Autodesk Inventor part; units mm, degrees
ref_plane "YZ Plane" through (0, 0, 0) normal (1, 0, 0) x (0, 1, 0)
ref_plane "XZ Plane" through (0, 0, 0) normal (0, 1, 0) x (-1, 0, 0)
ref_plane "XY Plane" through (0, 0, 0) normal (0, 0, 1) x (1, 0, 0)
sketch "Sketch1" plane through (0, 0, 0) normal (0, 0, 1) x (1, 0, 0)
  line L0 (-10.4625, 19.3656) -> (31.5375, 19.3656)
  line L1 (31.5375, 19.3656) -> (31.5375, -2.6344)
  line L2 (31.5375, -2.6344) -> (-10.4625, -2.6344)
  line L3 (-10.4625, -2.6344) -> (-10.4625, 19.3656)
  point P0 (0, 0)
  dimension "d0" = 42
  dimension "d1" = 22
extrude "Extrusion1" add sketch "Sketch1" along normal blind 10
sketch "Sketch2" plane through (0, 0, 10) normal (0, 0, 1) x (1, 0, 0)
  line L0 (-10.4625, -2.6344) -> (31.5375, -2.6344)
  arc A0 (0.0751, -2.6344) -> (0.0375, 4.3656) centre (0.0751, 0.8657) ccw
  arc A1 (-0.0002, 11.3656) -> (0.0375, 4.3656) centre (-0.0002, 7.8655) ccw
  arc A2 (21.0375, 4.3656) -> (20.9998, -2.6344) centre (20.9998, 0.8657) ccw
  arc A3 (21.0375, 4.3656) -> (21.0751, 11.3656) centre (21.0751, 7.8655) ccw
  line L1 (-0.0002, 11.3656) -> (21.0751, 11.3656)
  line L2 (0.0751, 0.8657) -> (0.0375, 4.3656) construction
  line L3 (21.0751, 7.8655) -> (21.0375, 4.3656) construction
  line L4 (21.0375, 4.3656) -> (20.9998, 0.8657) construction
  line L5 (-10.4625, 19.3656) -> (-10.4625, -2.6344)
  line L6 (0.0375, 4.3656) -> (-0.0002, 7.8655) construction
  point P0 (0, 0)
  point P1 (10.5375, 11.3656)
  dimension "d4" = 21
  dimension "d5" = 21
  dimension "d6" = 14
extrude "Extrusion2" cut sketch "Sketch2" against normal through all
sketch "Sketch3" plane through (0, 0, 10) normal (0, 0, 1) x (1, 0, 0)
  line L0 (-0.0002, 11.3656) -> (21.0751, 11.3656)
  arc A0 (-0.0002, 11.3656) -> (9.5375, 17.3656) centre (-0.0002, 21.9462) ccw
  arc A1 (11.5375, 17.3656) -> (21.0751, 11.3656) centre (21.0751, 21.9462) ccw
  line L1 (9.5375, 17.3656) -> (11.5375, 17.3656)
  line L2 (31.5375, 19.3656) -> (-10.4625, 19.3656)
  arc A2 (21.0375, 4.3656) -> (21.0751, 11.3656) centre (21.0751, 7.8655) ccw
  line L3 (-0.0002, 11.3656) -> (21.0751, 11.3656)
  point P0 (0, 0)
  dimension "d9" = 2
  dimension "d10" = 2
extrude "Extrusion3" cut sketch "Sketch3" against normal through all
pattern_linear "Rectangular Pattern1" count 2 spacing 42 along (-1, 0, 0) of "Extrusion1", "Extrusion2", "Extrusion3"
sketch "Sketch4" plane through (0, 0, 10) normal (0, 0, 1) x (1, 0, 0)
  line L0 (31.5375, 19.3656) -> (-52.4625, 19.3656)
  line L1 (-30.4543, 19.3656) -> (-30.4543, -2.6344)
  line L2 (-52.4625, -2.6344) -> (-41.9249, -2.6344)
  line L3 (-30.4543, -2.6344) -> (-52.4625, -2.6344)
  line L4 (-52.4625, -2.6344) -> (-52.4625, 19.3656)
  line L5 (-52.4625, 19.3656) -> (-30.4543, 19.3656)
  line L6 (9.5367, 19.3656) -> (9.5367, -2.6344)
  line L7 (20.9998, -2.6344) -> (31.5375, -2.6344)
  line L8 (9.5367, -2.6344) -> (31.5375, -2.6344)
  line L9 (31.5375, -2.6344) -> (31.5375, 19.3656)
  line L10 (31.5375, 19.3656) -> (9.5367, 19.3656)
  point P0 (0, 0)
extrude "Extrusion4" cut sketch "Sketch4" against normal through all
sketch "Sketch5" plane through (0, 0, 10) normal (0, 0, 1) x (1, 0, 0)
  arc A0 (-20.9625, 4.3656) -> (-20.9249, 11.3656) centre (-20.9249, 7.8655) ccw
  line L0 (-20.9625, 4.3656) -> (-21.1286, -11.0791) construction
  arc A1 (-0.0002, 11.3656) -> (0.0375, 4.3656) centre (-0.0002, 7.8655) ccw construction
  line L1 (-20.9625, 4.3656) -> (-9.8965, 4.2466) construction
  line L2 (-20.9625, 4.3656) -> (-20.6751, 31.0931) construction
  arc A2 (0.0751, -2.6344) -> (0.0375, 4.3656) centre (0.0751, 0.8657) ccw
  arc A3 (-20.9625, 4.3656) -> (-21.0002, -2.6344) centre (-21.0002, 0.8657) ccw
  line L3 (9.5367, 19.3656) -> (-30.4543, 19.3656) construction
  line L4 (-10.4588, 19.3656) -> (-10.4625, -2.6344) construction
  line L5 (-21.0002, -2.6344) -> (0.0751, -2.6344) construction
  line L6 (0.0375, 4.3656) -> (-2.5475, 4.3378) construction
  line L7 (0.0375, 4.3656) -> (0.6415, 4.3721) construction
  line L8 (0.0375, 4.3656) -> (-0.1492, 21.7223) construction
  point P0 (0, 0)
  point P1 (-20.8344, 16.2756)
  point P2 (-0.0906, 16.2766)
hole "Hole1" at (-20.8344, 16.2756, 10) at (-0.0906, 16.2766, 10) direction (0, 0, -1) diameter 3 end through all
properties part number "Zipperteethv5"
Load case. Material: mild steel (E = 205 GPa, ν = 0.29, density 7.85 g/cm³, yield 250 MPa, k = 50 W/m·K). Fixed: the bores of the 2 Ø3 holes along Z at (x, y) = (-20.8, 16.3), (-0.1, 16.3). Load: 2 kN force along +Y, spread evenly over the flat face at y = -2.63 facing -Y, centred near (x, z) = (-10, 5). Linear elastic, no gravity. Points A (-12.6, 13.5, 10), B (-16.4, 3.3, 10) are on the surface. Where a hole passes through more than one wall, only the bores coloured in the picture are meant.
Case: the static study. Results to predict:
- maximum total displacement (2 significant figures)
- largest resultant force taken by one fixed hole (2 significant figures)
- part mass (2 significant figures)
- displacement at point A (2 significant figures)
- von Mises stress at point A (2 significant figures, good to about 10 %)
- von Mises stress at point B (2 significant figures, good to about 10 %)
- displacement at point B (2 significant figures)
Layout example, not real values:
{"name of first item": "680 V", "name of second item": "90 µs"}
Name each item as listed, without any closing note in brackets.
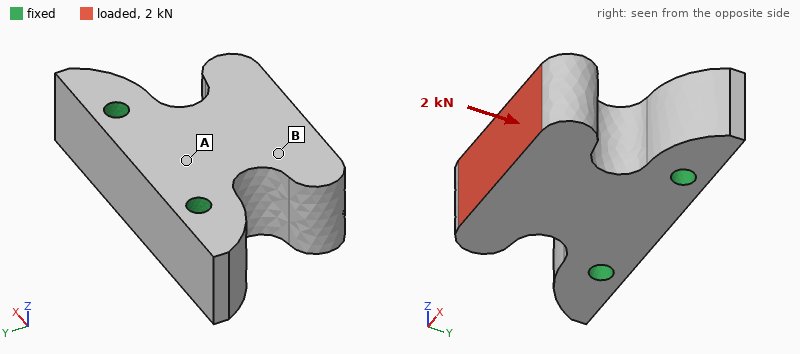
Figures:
{"maximum total displacement": "2.1 µm", "largest resultant force taken by one fixed hole": "1.1 kN", "part mass": "45 g", "displacement at point A": "1.1 µm", "von Mises stress at point A": "5.9 MPa", "von Mises stress at point B": "14 MPa", "displacement at point B": "1.5 µm"}
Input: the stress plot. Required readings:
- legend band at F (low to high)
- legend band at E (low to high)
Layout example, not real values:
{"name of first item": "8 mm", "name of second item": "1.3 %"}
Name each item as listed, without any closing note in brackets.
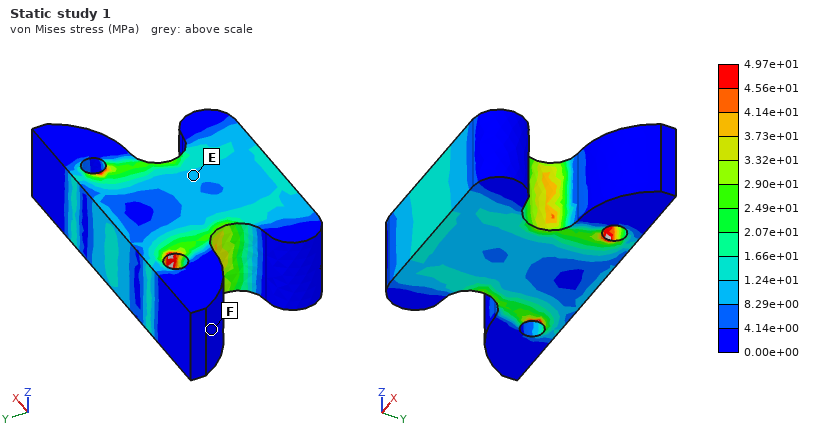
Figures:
{"legend band at F": "0.00e+00 to 4.14e+00 MPa", "legend band at E": "8.29e+00 to 1.24e+01 MPa"}
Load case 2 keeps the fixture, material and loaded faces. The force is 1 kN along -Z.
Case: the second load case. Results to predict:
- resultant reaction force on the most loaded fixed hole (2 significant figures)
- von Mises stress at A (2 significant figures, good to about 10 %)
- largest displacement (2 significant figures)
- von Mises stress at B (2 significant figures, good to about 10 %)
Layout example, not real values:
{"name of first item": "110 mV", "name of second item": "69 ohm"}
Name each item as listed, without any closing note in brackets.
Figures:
{"resultant reaction force on the most loaded fixed hole": "500 N", "von Mises stress at A": "31 MPa", "largest displacement": "16 µm", "von Mises stress at B": "20 MPa"}
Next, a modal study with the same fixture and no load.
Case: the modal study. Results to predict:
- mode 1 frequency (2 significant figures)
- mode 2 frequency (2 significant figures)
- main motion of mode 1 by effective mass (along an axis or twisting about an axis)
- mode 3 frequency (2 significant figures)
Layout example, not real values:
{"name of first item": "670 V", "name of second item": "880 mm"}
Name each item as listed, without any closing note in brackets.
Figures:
{"mode 1 frequency": "12 kHz", "mode 2 frequency": "21 kHz", "main motion of mode 1 by effective mass": "along Z", "mode 3 frequency": "22 kHz"}
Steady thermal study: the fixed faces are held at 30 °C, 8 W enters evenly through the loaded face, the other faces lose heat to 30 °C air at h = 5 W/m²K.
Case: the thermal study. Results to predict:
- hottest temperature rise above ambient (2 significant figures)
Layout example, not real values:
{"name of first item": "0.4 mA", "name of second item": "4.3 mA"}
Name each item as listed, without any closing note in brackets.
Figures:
{"hottest temperature rise above ambient": "20 K"}
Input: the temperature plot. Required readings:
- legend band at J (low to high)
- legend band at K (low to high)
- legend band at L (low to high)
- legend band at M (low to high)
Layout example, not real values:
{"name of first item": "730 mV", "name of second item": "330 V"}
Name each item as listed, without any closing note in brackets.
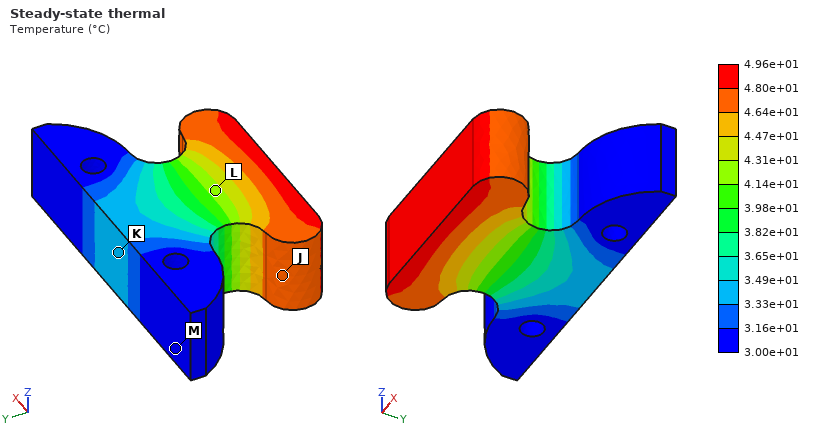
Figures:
{"legend band at J": "4.64e+01 to 4.80e+01 °C", "legend band at K": "3.33e+01 to 3.49e+01 °C", "legend band at L": "4.14e+01 to 4.31e+01 °C", "legend band at M": "3.00e+01 to 3.16e+01 °C"}
